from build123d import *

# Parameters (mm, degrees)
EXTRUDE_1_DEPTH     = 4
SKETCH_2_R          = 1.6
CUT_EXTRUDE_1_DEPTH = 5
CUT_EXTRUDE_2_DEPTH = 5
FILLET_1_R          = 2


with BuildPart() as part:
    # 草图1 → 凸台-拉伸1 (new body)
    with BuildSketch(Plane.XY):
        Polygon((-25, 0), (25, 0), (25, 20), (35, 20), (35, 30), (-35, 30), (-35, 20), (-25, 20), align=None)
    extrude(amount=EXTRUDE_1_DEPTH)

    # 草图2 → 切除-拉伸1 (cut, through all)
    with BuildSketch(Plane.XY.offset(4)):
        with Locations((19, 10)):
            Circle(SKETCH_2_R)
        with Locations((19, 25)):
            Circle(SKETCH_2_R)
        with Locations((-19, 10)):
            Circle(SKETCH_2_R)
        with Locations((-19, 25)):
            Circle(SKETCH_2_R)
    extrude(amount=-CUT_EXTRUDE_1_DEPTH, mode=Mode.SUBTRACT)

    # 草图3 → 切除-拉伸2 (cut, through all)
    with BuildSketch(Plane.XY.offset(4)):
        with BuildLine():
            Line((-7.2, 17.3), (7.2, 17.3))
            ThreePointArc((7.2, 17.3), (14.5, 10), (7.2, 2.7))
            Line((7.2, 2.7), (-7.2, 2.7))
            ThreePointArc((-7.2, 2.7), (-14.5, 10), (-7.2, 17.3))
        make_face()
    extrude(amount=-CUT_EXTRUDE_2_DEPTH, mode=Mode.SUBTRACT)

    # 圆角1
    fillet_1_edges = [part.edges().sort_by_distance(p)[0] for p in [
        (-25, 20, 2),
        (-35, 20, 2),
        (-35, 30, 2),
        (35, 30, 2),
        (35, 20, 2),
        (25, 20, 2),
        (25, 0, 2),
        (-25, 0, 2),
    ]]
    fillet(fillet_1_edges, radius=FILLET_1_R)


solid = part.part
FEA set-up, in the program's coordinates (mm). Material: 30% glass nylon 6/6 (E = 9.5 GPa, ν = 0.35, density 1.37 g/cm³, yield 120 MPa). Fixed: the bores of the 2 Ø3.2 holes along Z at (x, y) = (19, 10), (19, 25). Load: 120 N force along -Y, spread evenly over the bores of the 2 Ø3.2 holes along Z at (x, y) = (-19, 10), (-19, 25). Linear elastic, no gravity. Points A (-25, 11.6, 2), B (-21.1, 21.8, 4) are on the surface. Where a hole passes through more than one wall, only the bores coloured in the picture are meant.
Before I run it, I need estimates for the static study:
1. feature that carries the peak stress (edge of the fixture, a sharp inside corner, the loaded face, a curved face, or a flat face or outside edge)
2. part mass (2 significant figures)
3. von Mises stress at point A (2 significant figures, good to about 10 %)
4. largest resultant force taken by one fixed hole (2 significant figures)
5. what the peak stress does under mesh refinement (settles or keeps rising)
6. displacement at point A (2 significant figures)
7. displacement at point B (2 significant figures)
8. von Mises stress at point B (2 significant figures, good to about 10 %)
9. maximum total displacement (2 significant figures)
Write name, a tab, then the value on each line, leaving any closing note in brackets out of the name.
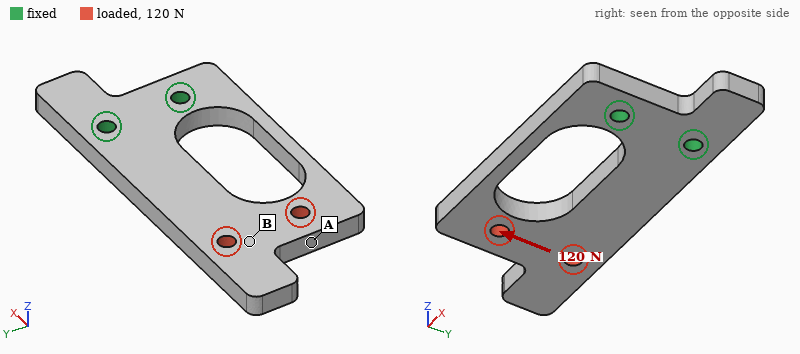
feature that carries the peak stress	edge of the fixture
part mass	7.1 g
von Mises stress at point A	8.9 MPa
largest resultant force taken by one fixed hole	280 N
what the peak stress does under mesh refinement	keeps rising
displacement at point A	0.15 mm
displacement at point B	0.15 mm
von Mises stress at point B	3.3 MPa
maximum total displacement	0.20 mm
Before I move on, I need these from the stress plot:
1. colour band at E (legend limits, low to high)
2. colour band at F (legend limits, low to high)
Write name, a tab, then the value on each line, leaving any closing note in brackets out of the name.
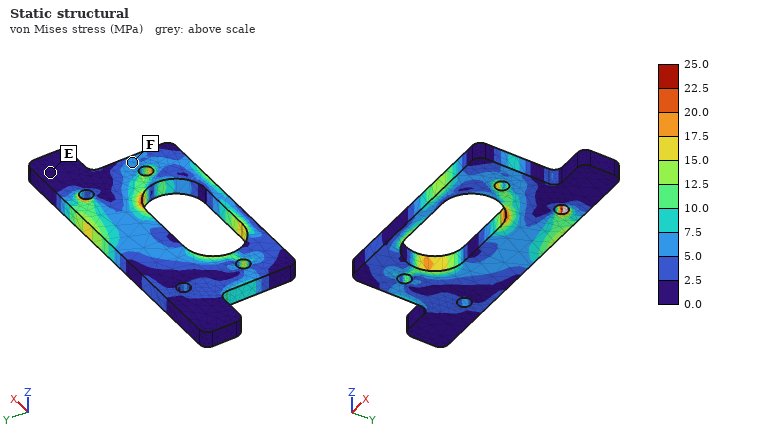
colour band at E	0.0 to 2.5 MPa
colour band at F	5.0 to 7.5 MPa
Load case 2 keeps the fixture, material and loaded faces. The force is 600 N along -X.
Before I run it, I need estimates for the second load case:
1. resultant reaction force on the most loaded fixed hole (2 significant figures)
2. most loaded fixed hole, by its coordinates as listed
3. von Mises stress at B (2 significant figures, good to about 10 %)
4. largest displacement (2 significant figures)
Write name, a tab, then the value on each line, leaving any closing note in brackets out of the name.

resultant reaction force on the most loaded fixed hole	340 N
most loaded fixed hole, by its coordinates as listed	(19, 25)
von Mises stress at B	4.2 MPa
largest displacement	96 µm
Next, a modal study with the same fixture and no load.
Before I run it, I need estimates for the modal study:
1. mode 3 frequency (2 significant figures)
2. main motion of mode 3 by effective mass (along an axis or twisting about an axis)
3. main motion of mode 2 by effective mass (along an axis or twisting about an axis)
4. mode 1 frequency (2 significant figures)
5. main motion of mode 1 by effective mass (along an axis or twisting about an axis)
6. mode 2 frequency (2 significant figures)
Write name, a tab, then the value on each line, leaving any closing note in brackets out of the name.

mode 3 frequency	2500 Hz
main motion of mode 3 by effective mass	along Y
main motion of mode 2 by effective mass	twisting about X
mode 1 frequency	600 Hz
main motion of mode 1 by effective mass	along Z
mode 2 frequency	1900 Hz
